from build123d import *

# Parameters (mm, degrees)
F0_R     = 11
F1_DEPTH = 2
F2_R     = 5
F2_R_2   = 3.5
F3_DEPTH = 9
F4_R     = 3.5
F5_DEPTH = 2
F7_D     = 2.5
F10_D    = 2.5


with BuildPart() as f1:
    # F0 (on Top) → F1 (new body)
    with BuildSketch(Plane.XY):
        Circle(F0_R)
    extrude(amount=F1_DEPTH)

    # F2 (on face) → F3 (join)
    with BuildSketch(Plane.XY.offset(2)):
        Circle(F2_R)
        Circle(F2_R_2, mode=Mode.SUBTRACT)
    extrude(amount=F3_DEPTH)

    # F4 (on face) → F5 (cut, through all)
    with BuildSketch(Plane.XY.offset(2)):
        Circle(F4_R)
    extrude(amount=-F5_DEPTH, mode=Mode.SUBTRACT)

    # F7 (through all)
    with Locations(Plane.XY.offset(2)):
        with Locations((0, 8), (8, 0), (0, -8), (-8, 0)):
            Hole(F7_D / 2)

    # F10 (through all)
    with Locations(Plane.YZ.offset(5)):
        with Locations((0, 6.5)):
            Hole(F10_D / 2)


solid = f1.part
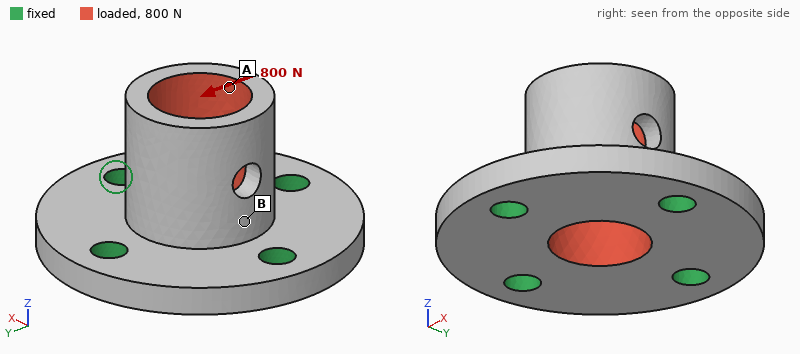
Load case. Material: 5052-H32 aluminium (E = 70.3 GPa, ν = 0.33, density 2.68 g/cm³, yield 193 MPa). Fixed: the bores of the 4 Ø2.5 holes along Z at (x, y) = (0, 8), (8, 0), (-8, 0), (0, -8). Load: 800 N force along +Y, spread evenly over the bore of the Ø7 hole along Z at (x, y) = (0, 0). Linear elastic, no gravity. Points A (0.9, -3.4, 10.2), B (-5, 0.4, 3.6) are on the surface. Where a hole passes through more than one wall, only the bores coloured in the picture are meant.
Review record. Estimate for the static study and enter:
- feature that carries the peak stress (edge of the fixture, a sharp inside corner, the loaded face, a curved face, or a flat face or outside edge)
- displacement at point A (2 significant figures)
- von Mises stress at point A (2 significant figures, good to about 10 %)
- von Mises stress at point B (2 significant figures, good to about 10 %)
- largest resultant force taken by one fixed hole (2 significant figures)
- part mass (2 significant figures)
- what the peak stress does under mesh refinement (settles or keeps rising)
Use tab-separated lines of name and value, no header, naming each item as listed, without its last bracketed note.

feature that carries the peak stress	edge of the fixture
displacement at point A	18 µm
von Mises stress at point A	12 MPa
von Mises stress at point B	36 MPa
largest resultant force taken by one fixed hole	360 N
part mass	2.7 g
what the peak stress does under mesh refinement	keeps rising
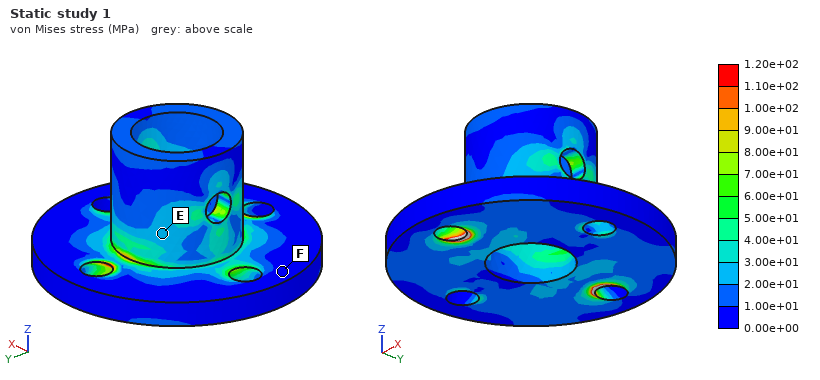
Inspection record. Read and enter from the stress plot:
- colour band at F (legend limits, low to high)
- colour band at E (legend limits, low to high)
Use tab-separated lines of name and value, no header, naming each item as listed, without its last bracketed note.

colour band at F	0.00e+00 to 1.00e+01 MPa
colour band at E	2.00e+01 to 3.00e+01 MPa
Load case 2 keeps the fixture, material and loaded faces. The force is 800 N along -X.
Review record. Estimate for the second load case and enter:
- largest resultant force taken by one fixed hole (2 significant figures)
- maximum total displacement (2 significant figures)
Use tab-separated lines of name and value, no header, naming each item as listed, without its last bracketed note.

largest resultant force taken by one fixed hole	360 N
maximum total displacement	19 µm
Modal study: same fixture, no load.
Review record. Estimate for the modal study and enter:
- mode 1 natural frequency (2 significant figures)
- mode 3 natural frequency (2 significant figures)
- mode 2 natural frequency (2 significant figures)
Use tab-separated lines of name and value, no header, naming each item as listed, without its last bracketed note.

mode 1 natural frequency	34 kHz
mode 3 natural frequency	55 kHz
mode 2 natural frequency	35 kHz
